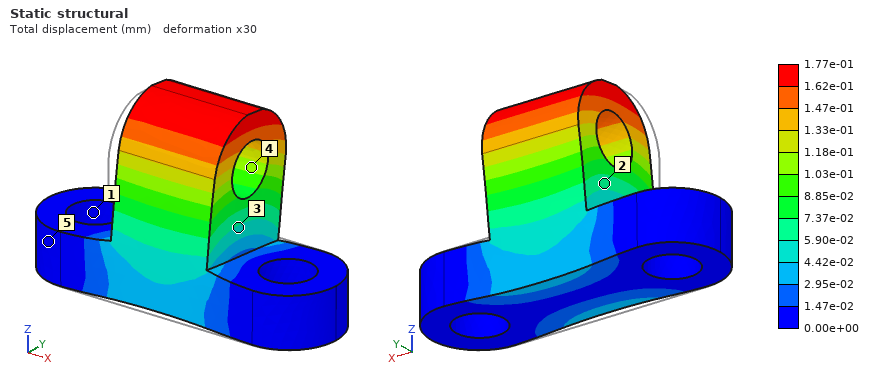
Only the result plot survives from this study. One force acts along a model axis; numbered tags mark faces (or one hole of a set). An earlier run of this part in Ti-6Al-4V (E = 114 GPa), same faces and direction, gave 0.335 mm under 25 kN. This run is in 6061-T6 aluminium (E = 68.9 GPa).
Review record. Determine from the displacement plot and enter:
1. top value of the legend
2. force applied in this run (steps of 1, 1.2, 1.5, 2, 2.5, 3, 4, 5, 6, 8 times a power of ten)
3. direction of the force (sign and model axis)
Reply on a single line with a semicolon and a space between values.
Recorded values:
1.77e-01 mm; 8 kN; +Y
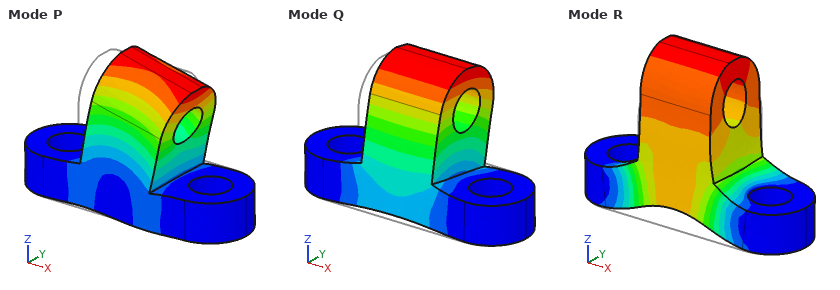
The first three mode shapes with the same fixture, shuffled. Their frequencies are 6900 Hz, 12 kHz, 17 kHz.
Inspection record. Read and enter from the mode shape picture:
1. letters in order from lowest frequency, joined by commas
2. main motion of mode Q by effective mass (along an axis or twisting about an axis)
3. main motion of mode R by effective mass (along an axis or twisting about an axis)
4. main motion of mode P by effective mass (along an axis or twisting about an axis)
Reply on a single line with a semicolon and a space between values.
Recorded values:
Q, P, R; along Y; along Z; along X
